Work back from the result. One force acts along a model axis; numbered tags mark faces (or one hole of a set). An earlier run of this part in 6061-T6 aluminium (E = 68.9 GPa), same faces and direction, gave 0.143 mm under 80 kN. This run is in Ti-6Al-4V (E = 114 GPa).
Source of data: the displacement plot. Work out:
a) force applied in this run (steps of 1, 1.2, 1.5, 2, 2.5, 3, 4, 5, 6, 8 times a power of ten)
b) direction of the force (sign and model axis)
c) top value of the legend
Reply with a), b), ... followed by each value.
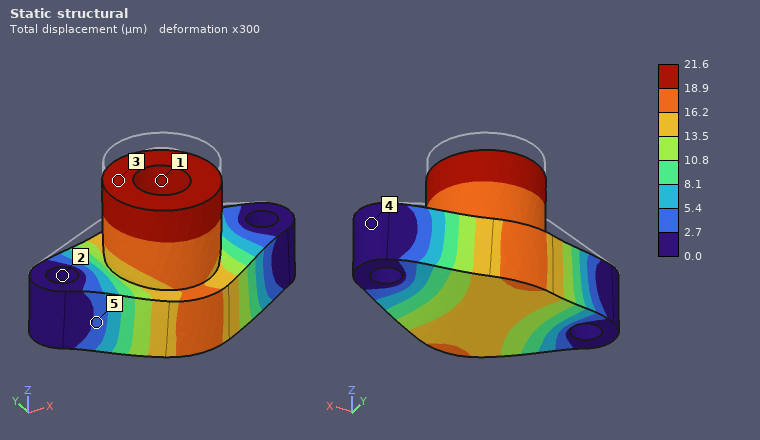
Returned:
a) 20 kN
b) -Z
c) 21.6 µm
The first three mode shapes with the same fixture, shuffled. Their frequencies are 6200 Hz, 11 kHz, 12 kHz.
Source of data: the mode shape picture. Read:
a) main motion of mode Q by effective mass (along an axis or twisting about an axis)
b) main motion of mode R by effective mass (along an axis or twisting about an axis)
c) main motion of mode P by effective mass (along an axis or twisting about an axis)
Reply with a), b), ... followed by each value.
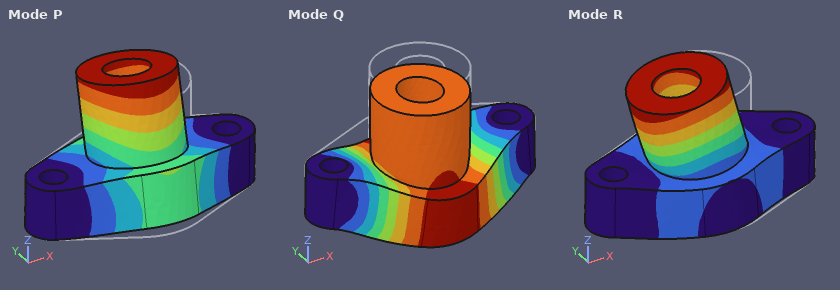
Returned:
a) along Z
b) along X
c) along Y
